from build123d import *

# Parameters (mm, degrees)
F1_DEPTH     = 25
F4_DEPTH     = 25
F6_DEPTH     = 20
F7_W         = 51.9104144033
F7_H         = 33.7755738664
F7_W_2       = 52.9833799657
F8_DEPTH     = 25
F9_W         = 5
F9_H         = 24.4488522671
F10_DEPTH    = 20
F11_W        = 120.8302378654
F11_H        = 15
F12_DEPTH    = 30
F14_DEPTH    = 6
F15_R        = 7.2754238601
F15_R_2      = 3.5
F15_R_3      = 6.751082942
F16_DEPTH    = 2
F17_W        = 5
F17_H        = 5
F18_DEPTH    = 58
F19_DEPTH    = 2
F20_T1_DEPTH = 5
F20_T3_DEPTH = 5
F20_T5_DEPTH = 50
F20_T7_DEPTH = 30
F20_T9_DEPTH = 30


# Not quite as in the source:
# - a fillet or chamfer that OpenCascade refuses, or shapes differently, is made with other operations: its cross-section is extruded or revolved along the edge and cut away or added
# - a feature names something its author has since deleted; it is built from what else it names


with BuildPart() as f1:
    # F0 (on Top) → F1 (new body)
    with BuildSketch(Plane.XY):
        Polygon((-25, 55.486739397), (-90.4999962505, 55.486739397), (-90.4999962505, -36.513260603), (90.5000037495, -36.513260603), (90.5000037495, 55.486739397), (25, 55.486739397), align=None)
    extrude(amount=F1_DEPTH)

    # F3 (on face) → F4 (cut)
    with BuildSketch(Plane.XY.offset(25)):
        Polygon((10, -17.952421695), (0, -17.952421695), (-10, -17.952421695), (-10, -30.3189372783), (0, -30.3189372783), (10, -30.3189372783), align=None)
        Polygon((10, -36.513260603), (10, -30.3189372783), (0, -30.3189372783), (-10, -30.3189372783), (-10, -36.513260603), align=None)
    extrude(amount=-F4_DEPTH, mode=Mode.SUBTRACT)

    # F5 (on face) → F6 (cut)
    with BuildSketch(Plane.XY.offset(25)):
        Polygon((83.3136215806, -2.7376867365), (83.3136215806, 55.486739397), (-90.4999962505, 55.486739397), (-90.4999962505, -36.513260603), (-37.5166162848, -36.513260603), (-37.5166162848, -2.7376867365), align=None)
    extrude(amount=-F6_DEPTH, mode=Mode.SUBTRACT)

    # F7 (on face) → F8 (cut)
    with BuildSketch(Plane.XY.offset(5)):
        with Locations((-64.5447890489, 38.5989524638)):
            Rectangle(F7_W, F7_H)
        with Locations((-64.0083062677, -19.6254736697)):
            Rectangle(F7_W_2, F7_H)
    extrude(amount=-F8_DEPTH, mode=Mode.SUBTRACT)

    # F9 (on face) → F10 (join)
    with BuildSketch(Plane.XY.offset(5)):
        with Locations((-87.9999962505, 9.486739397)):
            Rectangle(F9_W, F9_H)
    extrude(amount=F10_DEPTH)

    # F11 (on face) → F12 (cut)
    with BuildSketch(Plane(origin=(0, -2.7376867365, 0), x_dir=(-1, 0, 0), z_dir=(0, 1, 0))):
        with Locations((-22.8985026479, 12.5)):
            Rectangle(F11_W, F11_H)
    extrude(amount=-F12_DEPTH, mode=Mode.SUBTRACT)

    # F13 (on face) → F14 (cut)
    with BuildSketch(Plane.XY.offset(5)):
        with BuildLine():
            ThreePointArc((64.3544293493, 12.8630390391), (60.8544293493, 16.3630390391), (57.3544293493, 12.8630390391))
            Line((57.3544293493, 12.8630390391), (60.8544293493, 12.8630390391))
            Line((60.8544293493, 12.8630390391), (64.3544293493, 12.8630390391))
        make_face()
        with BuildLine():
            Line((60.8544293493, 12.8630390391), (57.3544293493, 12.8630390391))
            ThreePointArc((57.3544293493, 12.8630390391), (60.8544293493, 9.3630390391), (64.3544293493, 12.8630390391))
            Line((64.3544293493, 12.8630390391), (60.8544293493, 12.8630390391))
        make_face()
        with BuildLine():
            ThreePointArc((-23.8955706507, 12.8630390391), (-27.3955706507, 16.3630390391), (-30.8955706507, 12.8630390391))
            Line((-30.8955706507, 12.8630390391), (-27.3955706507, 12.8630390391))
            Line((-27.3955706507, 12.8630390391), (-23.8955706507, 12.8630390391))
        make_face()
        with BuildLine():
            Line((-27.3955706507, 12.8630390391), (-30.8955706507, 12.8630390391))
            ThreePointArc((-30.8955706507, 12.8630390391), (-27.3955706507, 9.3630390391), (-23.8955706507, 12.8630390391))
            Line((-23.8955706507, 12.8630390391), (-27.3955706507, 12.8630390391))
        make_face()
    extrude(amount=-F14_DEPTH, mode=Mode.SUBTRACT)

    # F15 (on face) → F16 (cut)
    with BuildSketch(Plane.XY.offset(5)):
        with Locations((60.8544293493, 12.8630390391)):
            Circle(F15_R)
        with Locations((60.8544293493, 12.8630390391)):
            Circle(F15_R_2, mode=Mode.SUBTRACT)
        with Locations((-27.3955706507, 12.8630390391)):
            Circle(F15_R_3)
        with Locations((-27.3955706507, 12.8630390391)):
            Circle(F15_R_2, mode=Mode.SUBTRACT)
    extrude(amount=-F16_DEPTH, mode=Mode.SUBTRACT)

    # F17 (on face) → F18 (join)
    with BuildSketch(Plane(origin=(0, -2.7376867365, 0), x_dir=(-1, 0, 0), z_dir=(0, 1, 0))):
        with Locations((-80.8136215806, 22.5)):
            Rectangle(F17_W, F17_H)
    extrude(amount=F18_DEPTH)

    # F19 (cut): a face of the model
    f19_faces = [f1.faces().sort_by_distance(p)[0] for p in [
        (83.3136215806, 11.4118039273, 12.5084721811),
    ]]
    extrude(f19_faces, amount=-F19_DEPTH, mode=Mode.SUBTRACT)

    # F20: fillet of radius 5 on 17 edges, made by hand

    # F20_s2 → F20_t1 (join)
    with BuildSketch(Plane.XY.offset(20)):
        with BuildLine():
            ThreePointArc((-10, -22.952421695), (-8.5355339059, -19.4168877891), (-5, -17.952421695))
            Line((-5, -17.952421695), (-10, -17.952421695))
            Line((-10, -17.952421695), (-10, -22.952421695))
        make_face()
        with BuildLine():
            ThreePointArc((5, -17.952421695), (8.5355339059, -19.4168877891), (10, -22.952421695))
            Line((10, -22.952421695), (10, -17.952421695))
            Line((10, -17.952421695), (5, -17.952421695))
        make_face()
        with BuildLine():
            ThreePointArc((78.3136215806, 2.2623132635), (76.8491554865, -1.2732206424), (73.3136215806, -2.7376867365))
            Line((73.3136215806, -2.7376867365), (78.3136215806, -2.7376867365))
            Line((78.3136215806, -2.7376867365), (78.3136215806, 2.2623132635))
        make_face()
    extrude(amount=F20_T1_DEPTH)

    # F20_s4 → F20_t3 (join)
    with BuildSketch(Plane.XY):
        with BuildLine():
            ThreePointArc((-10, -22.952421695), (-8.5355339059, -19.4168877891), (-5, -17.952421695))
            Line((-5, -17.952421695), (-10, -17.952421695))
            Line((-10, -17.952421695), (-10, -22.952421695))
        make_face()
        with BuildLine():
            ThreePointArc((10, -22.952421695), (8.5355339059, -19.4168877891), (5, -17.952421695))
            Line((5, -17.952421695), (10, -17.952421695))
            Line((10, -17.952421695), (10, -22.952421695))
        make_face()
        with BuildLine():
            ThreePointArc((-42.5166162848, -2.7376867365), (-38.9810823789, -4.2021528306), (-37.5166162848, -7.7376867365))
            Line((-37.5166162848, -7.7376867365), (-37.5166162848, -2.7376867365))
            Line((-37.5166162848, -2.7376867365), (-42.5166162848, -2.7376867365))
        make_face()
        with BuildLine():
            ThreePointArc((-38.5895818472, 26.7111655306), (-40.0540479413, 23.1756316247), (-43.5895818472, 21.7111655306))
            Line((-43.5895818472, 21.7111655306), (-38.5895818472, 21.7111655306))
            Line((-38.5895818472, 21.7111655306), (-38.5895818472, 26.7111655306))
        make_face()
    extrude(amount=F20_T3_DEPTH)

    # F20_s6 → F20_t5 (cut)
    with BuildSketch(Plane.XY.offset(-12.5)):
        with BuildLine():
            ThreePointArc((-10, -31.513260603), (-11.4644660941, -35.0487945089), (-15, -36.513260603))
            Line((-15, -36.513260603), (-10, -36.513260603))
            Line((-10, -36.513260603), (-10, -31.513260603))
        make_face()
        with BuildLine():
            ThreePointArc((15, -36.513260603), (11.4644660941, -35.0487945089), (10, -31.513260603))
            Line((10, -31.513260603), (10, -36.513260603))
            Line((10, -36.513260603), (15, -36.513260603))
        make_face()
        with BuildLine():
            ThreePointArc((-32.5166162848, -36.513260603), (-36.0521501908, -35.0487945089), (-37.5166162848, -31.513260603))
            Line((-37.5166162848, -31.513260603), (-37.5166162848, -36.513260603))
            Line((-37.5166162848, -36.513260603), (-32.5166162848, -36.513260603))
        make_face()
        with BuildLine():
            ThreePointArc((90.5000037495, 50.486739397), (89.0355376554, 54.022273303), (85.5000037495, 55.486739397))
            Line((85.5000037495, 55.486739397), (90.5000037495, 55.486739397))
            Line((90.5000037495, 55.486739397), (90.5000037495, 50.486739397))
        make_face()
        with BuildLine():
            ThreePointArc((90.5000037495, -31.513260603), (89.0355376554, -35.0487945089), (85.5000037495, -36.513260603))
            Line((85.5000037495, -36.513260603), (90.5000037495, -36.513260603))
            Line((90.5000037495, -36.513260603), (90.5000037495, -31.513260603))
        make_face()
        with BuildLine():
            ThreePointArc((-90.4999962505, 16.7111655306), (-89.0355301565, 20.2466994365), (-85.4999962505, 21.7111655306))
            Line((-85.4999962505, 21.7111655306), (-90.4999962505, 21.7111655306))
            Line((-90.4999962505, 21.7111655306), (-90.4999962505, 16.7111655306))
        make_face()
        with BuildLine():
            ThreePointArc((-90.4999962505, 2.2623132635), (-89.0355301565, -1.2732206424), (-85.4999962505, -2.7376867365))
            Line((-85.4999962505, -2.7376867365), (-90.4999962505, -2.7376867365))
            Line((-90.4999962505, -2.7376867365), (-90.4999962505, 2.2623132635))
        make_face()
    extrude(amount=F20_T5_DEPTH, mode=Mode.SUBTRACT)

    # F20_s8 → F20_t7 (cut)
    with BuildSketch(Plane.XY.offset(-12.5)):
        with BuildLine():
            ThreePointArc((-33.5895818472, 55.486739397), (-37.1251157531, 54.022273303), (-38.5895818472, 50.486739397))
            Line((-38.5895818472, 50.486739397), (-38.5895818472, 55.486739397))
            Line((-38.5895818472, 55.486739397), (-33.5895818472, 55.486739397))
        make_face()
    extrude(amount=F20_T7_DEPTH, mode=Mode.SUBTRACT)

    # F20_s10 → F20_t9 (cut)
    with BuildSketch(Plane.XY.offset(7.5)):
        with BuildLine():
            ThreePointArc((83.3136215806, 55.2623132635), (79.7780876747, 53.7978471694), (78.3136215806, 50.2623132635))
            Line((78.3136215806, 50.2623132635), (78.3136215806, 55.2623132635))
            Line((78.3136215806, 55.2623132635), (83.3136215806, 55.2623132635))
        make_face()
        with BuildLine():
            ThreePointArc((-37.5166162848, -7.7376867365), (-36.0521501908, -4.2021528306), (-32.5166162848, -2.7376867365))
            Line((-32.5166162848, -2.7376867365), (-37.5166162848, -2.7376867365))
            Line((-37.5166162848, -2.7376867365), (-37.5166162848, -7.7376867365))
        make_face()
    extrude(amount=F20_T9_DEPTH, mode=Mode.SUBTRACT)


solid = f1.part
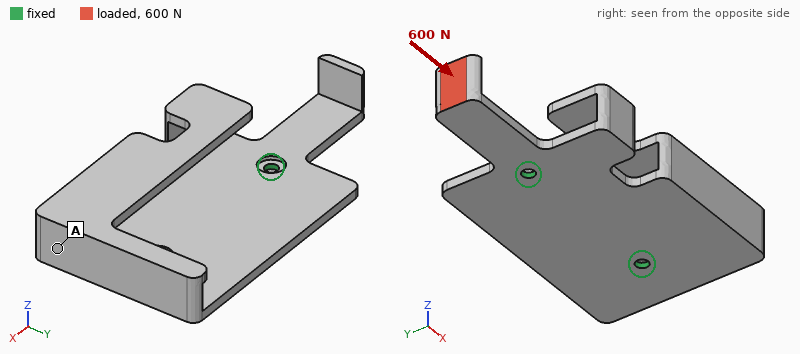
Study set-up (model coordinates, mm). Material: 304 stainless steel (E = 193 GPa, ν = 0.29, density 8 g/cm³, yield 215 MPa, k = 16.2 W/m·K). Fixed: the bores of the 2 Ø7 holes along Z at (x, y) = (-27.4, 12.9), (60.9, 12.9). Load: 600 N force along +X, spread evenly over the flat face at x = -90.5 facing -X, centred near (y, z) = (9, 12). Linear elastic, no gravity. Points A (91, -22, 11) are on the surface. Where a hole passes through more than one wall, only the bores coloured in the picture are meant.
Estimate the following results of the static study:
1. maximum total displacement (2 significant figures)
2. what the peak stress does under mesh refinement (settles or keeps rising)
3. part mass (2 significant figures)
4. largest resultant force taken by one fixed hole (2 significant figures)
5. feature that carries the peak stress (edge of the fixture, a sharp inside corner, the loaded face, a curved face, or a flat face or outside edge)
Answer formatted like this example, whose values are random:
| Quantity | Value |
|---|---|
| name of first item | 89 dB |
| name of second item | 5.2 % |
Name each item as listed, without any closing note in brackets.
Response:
| Quantity | Value |
|---|---|
| maximum total displacement | 0.30 mm |
| what the peak stress does under mesh refinement | keeps rising |
| part mass | 810 g |
| largest resultant force taken by one fixed hole | 300 N |
| feature that carries the peak stress | edge of the fixture |
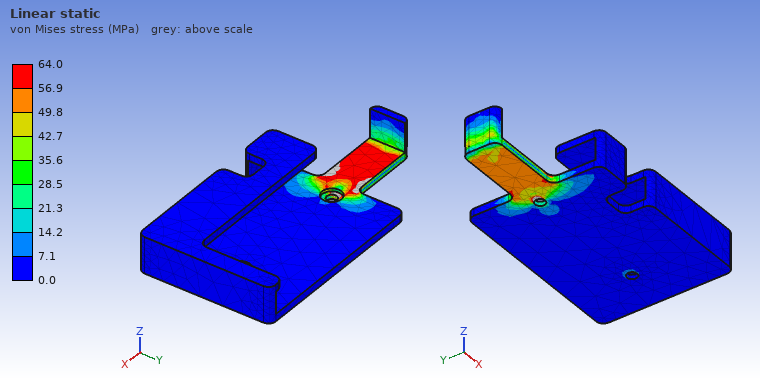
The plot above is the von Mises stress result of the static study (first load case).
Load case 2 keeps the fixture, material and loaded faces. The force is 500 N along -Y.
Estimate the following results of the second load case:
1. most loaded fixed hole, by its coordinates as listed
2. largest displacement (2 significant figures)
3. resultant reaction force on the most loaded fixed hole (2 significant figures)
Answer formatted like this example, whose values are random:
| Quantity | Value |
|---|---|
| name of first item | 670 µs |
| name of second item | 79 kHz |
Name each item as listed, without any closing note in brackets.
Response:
| Quantity | Value |
|---|---|
| most loaded fixed hole, by its coordinates as listed | (-27.4, 12.9) |
| largest displacement | 0.14 mm |
| resultant reaction force on the most loaded fixed hole | 820 N |
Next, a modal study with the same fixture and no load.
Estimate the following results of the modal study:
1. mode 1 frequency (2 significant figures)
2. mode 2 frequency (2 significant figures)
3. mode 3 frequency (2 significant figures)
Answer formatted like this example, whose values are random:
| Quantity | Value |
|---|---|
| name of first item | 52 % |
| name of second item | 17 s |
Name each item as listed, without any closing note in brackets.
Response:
| Quantity | Value |
|---|---|
| mode 1 frequency | 620 Hz |
| mode 2 frequency | 690 Hz |
| mode 3 frequency | 1000 Hz |
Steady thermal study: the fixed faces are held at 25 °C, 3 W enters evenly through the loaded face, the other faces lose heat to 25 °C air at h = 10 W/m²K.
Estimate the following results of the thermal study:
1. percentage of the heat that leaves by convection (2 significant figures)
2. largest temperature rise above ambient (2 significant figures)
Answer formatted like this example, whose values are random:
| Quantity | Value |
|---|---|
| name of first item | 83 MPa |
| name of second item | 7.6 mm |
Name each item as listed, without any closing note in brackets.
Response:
| Quantity | Value |
|---|---|
| percentage of the heat that leaves by convection | 59 % |
| largest temperature rise above ambient | 66 K |
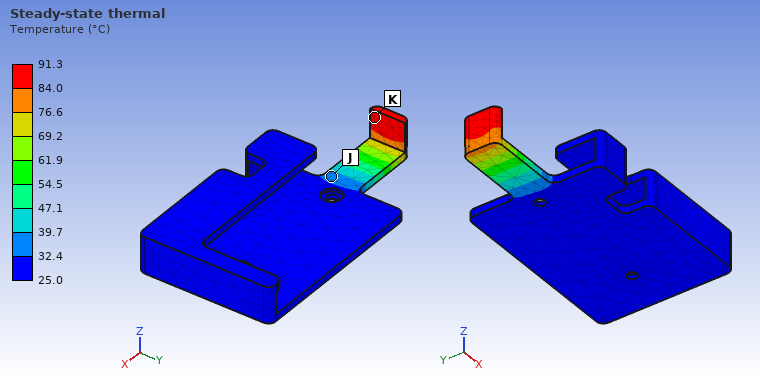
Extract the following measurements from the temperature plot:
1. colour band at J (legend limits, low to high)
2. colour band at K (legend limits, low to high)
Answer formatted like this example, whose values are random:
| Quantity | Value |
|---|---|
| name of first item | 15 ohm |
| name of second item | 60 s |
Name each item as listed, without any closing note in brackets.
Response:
| Quantity | Value |
|---|---|
| colour band at J | 32.4 to 39.7 °C |
| colour band at K | 84.0 to 91.3 °C |
